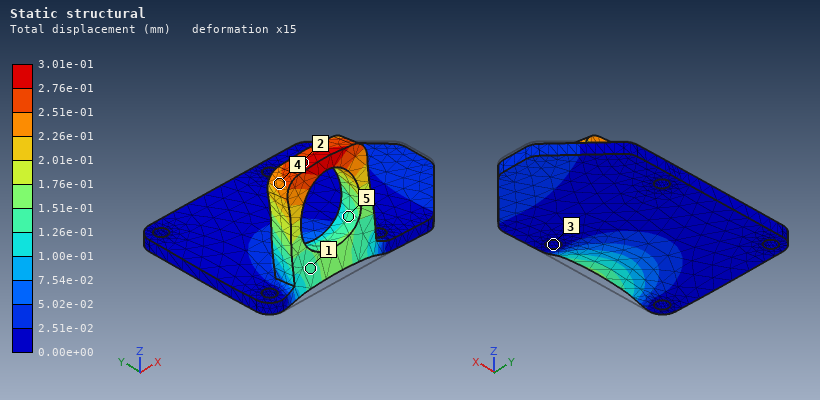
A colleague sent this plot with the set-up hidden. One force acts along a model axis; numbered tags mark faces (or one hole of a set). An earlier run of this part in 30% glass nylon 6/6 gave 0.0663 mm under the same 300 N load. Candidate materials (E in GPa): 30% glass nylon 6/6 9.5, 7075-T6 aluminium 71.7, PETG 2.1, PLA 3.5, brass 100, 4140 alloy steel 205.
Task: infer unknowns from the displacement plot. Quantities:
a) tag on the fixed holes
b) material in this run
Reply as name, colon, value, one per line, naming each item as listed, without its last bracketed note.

tag on the fixed holes: 3
material in this run: PETG
